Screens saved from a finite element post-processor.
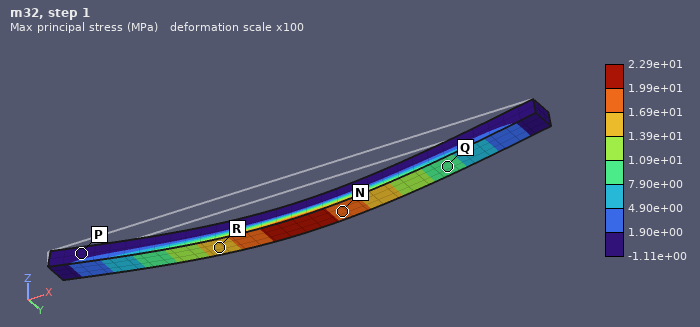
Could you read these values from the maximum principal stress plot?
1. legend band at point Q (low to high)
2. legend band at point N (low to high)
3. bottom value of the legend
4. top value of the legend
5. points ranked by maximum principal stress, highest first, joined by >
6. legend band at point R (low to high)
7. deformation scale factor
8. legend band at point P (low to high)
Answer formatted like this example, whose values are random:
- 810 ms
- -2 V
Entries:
- 7.90e+00 to 1.09e+01 MPa
- 1.69e+01 to 1.99e+01 MPa
- -1.11e+00 MPa
- 2.29e+01 MPa
- N > R > Q > P
- 1.39e+01 to 1.69e+01 MPa
- 100
- -1.11e+00 to 1.90e+00 MPa
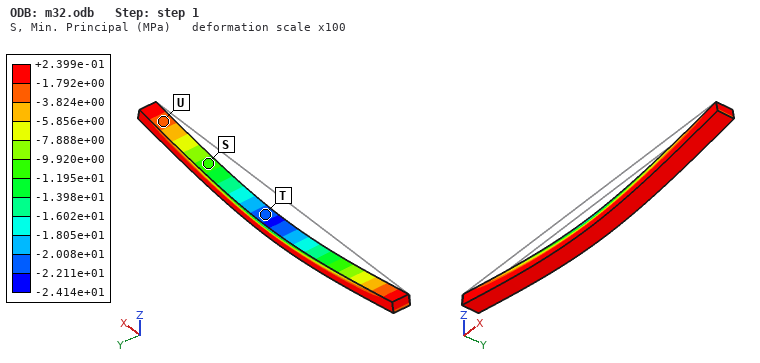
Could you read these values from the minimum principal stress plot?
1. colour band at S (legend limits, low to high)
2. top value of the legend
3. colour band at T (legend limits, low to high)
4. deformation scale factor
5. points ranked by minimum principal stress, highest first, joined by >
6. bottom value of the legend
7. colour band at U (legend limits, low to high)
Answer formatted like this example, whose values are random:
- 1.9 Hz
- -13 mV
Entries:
- -1.195e+01 to -9.920e+00 MPa
- +2.399e-01 MPa
- -2.211e+01 to -2.008e+01 MPa
- 100
- U > S > T
- -2.414e+01 MPa
- -3.824e+00 to -1.792e+00 MPa
